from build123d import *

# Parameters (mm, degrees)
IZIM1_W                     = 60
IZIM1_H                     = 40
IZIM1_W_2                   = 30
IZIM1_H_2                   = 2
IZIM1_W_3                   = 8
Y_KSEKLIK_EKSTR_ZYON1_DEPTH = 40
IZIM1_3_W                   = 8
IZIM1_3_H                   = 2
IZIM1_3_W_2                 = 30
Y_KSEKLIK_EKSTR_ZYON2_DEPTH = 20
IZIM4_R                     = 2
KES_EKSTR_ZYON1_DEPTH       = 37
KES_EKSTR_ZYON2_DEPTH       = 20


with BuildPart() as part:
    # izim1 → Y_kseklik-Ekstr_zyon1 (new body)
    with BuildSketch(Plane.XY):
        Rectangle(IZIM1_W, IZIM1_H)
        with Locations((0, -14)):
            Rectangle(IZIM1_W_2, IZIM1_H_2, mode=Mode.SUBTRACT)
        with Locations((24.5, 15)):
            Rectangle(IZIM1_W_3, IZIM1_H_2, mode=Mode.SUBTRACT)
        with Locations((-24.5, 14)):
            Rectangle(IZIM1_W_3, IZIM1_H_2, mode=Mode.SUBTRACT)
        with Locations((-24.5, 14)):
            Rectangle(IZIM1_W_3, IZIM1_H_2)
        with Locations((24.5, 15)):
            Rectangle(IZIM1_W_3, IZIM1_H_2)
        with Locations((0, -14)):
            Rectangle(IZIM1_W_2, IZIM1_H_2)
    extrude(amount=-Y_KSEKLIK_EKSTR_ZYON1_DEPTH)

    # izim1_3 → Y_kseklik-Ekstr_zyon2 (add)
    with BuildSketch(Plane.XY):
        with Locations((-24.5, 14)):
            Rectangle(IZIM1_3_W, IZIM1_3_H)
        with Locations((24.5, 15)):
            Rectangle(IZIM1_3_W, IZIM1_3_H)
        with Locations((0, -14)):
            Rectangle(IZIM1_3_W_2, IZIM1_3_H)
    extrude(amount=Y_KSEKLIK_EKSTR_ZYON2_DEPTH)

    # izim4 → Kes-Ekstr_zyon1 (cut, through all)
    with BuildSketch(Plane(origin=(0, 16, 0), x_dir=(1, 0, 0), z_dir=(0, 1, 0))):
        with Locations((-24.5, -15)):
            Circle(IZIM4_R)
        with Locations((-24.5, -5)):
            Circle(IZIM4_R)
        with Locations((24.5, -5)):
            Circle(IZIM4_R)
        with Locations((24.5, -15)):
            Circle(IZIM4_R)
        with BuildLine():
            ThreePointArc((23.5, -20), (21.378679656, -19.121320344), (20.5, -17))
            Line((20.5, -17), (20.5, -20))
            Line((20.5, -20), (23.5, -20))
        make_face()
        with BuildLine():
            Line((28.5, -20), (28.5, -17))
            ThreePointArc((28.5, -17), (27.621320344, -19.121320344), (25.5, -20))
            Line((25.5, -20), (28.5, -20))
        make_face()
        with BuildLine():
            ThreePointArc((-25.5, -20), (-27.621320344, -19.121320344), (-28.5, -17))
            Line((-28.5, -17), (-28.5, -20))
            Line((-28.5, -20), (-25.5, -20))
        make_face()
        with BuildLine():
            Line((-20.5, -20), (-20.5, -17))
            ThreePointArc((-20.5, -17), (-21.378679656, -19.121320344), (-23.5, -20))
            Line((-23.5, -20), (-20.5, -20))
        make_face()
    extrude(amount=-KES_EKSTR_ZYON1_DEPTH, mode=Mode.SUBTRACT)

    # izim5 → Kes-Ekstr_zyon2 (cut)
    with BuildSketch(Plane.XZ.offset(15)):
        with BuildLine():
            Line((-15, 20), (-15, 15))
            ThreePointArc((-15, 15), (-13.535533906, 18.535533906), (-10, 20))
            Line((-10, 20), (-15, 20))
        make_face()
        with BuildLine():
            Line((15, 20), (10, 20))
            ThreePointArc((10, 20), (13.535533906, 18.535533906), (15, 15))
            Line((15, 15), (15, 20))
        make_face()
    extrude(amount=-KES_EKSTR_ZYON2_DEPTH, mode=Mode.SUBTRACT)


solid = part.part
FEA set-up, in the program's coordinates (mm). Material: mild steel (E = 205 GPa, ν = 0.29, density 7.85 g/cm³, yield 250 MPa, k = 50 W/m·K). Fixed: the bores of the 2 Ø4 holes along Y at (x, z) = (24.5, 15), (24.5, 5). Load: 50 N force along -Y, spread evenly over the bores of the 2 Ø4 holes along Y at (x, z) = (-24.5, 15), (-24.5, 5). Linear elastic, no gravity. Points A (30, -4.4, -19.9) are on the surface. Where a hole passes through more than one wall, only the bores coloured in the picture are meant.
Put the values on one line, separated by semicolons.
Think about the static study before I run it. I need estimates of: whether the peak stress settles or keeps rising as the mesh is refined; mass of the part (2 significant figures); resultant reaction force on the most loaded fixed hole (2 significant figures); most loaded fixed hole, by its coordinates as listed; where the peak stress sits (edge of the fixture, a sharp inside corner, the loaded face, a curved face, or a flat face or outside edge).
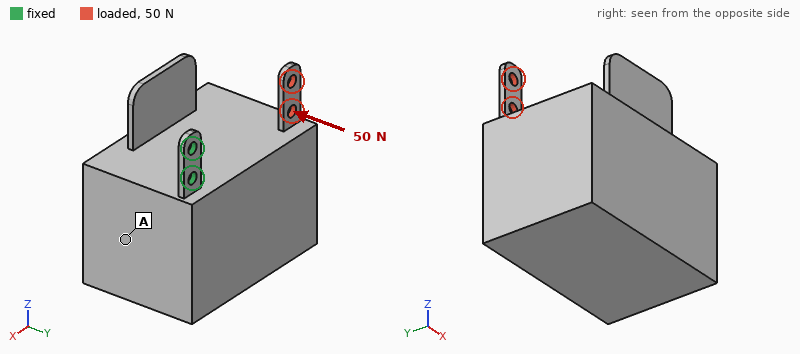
keeps rising; 770 g; 50 N; (24.5, 5); edge of the fixture
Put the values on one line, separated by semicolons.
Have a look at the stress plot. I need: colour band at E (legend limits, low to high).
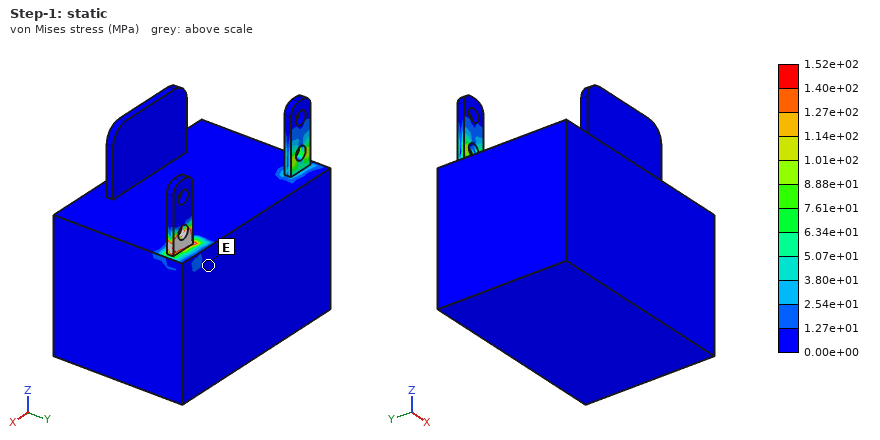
0.00e+00 to 1.27e+01 MPa
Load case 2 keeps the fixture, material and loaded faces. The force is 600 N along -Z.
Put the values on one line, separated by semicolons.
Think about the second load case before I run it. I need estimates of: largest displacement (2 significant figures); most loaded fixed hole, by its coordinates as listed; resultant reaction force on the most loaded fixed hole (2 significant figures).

0.85 mm; (24.5, 5); 810 N
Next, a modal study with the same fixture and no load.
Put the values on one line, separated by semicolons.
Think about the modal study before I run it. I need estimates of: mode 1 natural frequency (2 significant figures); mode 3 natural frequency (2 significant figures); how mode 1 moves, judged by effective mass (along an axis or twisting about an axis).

89 Hz; 300 Hz; along Y
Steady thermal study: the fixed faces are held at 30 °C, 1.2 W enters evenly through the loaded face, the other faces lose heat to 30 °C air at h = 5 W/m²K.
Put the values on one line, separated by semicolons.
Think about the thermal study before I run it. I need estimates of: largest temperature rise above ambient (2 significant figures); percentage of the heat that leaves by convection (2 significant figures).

29 K; 36 %
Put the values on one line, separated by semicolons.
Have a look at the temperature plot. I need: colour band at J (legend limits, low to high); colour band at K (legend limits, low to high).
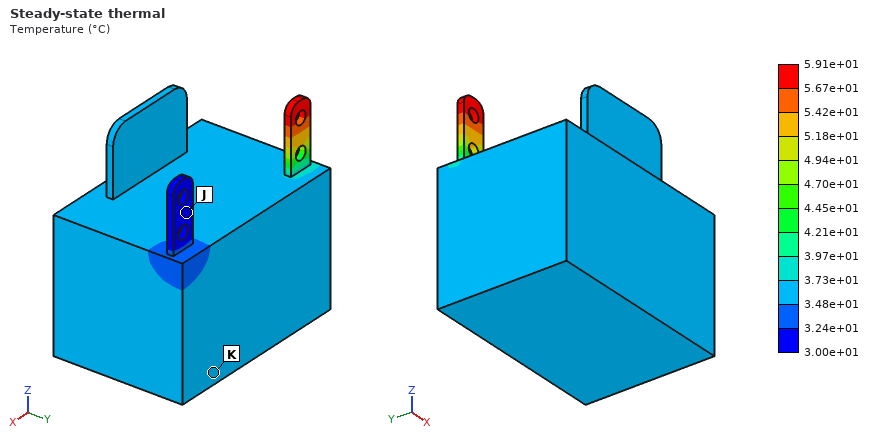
3.00e+01 to 3.24e+01 °C; 3.48e+01 to 3.73e+01 °C
